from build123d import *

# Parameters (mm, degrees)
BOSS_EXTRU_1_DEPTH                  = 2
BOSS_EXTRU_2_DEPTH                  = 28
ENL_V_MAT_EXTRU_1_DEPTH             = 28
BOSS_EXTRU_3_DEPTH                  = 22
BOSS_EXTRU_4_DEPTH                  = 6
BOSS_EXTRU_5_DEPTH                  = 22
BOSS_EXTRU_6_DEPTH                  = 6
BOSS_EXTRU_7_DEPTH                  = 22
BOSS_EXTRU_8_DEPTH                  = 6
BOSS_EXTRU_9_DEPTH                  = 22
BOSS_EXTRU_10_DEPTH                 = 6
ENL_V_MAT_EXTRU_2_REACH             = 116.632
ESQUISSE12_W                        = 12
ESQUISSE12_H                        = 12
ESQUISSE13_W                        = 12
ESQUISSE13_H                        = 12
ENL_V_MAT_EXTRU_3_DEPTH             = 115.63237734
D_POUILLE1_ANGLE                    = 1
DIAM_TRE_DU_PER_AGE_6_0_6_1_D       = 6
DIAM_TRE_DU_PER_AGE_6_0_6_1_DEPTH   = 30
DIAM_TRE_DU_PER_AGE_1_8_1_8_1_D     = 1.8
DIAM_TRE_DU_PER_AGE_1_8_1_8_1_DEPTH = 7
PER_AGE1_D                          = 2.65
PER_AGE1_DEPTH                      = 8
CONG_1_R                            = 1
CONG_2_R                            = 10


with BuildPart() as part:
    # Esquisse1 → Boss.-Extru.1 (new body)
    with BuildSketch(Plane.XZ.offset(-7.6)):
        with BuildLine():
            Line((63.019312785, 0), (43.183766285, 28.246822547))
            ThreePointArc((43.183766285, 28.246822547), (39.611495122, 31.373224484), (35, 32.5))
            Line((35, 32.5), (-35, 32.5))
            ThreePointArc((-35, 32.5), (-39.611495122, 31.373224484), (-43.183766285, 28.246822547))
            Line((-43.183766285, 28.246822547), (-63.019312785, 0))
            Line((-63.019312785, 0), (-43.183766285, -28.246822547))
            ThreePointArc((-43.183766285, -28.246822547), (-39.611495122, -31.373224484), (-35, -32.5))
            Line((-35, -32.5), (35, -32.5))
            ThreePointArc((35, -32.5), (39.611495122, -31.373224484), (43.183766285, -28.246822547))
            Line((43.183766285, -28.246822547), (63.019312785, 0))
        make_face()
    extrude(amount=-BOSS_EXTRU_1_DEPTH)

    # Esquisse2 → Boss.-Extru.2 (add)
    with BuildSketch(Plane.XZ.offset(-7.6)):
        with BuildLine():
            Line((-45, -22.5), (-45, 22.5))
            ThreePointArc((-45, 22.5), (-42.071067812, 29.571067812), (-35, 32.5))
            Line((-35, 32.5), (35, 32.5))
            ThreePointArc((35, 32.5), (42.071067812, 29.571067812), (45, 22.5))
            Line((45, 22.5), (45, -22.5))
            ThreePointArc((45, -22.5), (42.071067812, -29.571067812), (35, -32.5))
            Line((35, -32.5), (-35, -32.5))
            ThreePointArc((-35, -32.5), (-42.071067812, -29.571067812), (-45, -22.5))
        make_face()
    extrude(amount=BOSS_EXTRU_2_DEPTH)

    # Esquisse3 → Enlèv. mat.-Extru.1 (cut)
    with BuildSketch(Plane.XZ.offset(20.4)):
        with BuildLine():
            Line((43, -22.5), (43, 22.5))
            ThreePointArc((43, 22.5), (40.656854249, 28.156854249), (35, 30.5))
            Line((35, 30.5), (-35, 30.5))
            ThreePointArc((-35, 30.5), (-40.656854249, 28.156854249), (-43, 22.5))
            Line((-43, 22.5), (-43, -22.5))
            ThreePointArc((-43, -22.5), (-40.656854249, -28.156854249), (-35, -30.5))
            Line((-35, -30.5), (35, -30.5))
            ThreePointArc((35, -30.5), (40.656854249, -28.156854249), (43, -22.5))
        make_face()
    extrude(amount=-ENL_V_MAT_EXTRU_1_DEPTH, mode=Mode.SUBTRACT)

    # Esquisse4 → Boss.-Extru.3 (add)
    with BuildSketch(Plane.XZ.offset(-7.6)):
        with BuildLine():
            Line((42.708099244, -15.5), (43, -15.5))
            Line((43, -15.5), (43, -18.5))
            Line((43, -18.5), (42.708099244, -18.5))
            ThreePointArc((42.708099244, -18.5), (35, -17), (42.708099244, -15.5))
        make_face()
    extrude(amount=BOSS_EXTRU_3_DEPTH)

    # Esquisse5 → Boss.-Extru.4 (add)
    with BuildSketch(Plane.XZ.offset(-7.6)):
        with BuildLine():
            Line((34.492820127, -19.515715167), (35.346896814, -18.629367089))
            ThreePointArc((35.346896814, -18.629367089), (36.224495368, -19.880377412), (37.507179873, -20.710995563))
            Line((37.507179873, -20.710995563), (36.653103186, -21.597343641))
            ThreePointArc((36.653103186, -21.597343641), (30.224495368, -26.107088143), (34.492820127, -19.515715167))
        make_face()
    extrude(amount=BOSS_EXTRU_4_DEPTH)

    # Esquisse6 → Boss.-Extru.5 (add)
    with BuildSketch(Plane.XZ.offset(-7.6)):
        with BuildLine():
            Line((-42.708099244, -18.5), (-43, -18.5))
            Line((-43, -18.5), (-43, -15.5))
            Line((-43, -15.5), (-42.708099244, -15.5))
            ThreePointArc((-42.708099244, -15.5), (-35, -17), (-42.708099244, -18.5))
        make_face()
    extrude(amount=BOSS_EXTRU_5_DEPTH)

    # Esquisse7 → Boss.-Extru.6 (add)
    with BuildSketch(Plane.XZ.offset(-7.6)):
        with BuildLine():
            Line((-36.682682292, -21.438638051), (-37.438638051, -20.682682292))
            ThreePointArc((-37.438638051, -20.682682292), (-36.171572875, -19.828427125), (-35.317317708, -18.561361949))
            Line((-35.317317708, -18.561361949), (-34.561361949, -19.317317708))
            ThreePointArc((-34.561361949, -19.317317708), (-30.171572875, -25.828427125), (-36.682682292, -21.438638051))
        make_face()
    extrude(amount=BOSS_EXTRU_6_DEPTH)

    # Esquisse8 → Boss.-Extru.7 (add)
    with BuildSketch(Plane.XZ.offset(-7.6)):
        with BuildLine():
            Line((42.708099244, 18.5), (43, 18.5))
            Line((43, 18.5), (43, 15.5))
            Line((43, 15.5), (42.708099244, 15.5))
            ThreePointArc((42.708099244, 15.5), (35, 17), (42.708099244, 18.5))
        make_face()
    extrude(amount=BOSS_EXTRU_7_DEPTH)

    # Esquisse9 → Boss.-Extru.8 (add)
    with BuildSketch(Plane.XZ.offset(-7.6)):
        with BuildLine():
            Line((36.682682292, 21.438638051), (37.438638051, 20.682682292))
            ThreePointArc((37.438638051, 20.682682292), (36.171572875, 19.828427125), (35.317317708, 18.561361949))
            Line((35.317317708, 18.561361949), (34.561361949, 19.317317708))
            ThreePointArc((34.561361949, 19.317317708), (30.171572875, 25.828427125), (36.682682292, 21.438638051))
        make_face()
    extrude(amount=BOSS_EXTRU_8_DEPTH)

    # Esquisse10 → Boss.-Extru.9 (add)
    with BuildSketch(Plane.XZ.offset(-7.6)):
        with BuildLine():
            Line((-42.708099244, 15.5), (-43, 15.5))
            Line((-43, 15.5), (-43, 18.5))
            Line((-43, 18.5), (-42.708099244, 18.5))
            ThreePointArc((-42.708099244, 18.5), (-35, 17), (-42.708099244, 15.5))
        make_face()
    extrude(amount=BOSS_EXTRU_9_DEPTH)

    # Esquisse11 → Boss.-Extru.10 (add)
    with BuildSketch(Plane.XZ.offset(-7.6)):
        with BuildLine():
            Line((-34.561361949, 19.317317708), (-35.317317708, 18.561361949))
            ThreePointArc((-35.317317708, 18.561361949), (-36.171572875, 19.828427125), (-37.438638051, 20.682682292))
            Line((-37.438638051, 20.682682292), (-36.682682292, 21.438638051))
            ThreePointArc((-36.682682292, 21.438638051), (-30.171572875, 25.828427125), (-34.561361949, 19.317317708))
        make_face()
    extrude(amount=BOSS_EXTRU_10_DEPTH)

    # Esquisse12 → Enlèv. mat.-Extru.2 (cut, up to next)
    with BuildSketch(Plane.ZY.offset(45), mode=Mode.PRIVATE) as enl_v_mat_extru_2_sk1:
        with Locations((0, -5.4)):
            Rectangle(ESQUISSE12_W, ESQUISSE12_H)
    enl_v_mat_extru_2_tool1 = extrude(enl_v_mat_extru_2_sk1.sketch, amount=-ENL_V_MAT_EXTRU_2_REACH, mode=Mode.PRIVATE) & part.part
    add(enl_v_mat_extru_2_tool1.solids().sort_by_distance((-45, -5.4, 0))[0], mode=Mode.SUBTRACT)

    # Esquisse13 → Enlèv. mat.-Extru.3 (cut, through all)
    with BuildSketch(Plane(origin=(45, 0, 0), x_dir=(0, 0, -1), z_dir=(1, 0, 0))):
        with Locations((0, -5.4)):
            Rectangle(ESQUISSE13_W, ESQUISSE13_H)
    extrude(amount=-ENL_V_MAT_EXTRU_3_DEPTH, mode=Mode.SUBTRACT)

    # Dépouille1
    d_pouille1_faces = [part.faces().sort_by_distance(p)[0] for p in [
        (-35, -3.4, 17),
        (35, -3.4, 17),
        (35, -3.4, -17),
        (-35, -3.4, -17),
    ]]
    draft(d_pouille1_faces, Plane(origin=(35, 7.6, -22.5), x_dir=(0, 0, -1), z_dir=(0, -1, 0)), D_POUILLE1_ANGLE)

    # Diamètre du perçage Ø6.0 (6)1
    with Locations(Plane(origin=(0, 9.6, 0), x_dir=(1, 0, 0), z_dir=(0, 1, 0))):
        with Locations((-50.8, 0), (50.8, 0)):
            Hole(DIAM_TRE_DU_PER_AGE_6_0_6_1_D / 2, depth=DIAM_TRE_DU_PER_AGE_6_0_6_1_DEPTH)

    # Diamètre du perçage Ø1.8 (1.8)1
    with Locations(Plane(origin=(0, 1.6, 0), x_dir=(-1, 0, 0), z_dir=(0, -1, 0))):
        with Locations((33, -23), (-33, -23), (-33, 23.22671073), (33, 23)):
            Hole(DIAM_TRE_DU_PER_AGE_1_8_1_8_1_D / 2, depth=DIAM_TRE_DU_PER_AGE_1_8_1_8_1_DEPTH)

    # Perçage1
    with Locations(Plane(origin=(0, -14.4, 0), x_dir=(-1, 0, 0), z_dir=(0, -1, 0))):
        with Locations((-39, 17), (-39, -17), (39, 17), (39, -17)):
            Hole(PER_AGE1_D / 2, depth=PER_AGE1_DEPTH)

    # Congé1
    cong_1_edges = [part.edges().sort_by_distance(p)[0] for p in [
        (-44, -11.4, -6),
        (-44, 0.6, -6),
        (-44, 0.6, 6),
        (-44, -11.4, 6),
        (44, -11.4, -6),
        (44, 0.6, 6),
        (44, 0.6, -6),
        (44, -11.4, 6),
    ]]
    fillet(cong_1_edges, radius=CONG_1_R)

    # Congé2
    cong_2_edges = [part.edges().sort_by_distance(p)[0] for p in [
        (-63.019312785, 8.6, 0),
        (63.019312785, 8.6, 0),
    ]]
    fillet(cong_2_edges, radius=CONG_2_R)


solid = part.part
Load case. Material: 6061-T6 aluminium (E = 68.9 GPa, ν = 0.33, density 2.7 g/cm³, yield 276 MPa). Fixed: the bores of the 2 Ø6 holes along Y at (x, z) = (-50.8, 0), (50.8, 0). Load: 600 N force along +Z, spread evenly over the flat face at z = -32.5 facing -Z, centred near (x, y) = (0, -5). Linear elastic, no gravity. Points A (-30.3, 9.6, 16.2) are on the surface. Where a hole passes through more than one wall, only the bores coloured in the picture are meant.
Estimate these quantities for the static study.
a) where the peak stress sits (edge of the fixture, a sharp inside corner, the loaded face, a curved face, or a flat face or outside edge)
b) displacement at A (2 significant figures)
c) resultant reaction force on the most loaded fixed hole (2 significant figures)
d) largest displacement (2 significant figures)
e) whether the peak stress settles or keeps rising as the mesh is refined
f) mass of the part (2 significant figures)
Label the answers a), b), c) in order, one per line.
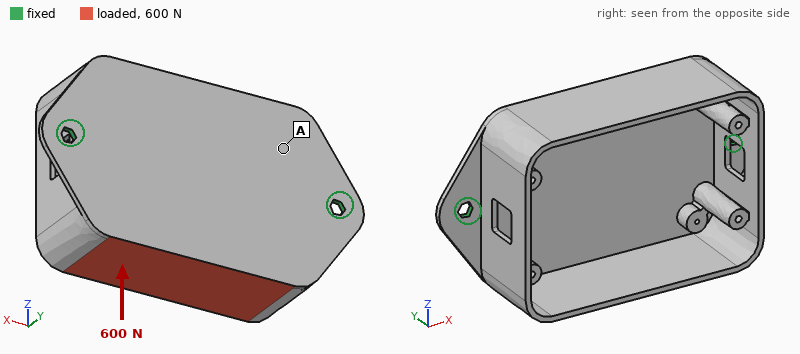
a) edge of the fixture
b) 0.10 mm
c) 300 N
d) 0.65 mm
e) keeps rising
f) 91 g
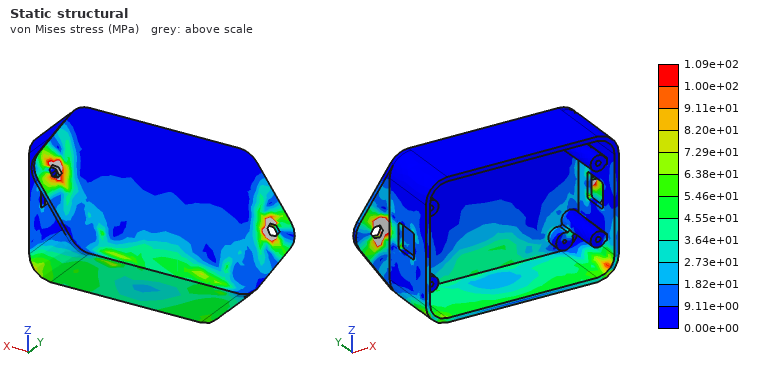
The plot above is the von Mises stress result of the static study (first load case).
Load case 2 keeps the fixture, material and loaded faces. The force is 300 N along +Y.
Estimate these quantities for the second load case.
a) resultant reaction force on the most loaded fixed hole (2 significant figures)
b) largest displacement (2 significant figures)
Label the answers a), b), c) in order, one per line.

a) 160 N
b) 0.36 mm
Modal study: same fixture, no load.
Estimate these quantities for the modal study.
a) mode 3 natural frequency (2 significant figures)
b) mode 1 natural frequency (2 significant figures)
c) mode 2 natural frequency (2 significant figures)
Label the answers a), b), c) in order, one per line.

a) 2300 Hz
b) 750 Hz
c) 1500 Hz
